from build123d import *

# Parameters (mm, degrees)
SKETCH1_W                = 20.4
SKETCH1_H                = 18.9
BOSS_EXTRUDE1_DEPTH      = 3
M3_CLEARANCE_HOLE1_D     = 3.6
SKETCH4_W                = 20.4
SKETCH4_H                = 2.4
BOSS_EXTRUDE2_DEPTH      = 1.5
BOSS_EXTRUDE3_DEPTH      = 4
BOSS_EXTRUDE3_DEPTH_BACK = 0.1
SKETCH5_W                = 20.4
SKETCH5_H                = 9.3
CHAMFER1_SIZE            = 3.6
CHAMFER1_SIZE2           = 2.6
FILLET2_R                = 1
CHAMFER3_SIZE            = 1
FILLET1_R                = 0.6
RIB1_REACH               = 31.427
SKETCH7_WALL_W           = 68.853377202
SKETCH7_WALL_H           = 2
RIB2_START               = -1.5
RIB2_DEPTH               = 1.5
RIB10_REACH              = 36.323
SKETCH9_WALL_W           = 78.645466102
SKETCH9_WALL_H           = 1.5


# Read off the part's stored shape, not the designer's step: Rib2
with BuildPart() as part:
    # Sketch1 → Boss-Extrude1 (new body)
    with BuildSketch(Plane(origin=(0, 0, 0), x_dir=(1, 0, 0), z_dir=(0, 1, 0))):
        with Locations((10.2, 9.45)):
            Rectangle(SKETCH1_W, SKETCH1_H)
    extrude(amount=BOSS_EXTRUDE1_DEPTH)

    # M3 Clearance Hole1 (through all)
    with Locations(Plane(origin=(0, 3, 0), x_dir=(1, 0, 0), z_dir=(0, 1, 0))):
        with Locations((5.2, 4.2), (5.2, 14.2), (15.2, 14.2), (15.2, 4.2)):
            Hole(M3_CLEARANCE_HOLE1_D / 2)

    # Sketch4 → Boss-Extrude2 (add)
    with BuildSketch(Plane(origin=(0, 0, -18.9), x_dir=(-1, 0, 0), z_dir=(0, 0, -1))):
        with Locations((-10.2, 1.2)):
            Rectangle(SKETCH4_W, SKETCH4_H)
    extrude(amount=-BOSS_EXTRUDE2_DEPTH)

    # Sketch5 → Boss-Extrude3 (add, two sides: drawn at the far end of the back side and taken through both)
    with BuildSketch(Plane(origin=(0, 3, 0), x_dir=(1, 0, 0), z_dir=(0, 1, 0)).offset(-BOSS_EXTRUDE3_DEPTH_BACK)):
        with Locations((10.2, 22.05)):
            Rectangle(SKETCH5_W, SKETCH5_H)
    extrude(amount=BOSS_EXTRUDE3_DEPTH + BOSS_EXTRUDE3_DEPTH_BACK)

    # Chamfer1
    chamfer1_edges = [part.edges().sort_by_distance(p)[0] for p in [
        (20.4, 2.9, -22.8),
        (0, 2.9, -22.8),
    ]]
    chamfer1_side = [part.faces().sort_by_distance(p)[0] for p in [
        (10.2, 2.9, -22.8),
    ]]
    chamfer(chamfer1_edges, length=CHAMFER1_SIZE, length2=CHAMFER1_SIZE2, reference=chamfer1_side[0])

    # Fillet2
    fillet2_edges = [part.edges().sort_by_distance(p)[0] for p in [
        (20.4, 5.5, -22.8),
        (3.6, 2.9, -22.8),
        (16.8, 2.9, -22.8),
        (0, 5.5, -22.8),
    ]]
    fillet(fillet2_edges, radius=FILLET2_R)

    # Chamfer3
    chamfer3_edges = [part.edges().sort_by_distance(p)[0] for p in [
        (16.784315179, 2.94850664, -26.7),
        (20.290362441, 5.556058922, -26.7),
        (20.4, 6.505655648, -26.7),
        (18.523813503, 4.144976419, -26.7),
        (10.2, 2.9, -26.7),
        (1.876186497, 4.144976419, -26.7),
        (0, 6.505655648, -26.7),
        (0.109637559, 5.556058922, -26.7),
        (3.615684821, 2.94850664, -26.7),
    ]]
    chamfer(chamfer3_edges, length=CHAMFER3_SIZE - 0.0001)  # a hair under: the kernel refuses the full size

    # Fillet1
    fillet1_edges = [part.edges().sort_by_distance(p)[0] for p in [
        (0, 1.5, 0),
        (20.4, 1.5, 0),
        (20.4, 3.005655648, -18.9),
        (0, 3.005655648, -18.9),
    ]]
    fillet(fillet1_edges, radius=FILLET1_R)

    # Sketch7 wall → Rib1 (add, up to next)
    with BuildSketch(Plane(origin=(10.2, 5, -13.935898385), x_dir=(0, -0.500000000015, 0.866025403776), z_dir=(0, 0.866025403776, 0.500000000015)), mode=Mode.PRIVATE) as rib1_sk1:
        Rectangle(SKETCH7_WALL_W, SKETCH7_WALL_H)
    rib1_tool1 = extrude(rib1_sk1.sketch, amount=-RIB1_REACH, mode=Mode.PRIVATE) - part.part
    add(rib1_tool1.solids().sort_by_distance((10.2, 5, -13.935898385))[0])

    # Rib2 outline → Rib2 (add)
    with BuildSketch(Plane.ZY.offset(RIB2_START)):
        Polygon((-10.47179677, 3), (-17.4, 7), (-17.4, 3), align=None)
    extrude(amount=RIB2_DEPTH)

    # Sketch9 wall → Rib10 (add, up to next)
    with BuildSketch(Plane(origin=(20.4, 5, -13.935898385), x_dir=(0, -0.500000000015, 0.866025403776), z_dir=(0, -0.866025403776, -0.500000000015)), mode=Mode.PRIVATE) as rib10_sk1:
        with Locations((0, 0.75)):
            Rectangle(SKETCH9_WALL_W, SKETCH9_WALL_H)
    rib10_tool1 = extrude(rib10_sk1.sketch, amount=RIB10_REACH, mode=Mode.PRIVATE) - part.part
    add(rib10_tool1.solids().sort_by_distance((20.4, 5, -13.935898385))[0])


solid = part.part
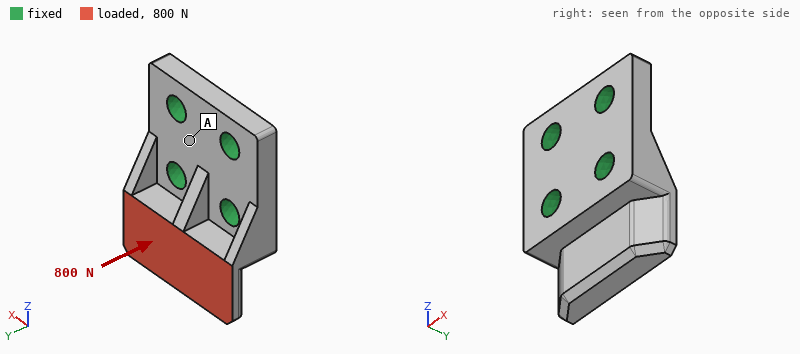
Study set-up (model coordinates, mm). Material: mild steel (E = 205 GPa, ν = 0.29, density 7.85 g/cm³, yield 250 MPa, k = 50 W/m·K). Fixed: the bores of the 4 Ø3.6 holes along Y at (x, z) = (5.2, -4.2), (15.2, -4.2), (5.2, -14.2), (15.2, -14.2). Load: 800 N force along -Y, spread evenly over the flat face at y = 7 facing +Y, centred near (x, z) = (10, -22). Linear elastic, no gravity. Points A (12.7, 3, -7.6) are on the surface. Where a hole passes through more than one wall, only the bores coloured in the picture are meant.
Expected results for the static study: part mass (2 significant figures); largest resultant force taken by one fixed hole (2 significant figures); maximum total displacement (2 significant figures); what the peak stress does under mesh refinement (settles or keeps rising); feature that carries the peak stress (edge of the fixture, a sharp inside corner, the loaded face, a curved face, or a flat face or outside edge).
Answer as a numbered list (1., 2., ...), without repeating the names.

1. 14 g
2. 490 N
3. 20 µm
4. keeps rising
5. edge of the fixture
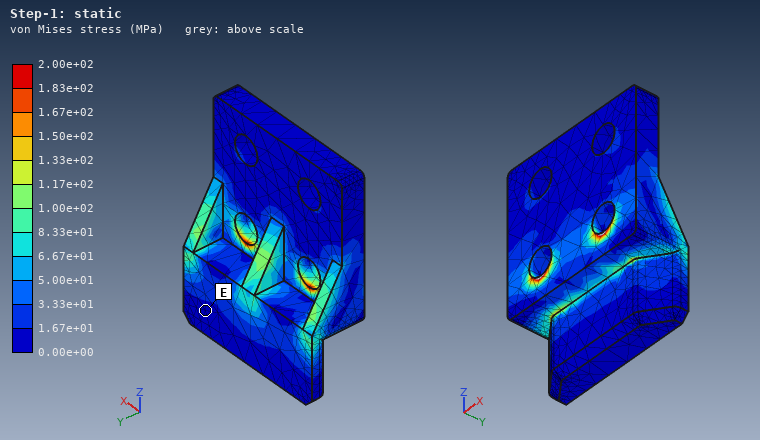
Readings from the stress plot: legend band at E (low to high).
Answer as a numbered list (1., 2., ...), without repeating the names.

1. 0.00e+00 to 1.67e+01 MPa
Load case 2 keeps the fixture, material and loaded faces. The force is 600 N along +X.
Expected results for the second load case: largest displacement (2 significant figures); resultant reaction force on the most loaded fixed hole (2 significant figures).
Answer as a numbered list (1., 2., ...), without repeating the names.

1. 3.7 µm
2. 480 N
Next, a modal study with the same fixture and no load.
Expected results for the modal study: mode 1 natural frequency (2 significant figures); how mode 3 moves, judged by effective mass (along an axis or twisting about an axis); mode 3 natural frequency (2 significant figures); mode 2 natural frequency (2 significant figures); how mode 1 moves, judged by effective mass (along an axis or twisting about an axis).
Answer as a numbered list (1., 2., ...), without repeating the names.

1. 16 kHz
2. along X
3. 39 kHz
4. 29 kHz
5. along Y
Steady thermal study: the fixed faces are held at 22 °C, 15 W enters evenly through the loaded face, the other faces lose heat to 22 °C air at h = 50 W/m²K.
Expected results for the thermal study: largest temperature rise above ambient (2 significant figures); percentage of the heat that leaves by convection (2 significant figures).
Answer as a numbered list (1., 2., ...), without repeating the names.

1. 43 K
2. 5.0 %
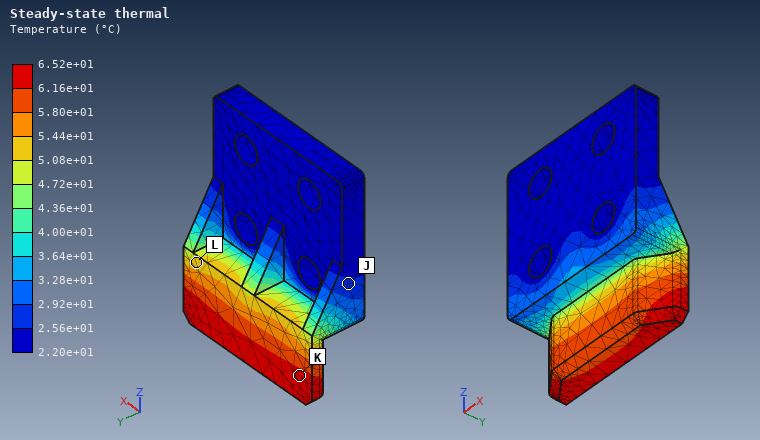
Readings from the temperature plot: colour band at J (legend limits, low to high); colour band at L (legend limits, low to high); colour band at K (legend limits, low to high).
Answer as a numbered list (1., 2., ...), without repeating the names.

1. 2.56e+01 to 2.92e+01 °C
2. 5.08e+01 to 5.44e+01 °C
3. 6.16e+01 to 6.52e+01 °C
